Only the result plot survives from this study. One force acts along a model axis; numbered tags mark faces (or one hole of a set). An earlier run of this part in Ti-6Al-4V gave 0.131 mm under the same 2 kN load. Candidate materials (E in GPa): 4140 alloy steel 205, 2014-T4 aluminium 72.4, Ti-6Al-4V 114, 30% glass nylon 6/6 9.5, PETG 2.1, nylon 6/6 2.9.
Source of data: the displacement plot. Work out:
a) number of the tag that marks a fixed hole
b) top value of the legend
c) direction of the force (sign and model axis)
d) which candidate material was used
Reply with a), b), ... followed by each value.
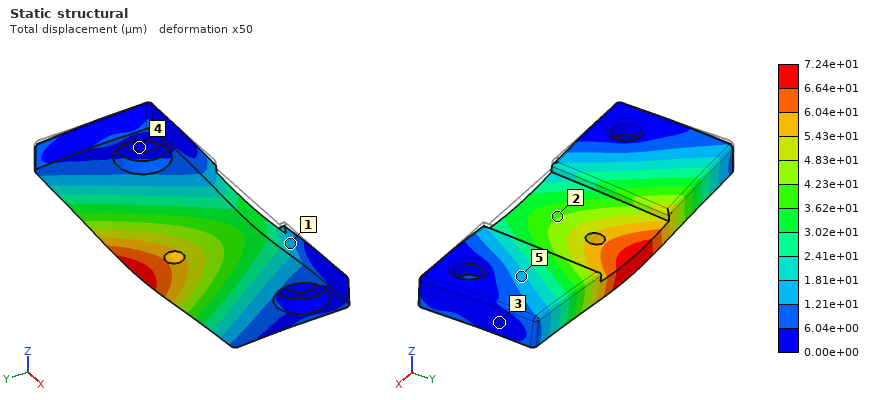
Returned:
a) 4
b) 7.24e+01 µm
c) -Z
d) 4140 alloy steel
